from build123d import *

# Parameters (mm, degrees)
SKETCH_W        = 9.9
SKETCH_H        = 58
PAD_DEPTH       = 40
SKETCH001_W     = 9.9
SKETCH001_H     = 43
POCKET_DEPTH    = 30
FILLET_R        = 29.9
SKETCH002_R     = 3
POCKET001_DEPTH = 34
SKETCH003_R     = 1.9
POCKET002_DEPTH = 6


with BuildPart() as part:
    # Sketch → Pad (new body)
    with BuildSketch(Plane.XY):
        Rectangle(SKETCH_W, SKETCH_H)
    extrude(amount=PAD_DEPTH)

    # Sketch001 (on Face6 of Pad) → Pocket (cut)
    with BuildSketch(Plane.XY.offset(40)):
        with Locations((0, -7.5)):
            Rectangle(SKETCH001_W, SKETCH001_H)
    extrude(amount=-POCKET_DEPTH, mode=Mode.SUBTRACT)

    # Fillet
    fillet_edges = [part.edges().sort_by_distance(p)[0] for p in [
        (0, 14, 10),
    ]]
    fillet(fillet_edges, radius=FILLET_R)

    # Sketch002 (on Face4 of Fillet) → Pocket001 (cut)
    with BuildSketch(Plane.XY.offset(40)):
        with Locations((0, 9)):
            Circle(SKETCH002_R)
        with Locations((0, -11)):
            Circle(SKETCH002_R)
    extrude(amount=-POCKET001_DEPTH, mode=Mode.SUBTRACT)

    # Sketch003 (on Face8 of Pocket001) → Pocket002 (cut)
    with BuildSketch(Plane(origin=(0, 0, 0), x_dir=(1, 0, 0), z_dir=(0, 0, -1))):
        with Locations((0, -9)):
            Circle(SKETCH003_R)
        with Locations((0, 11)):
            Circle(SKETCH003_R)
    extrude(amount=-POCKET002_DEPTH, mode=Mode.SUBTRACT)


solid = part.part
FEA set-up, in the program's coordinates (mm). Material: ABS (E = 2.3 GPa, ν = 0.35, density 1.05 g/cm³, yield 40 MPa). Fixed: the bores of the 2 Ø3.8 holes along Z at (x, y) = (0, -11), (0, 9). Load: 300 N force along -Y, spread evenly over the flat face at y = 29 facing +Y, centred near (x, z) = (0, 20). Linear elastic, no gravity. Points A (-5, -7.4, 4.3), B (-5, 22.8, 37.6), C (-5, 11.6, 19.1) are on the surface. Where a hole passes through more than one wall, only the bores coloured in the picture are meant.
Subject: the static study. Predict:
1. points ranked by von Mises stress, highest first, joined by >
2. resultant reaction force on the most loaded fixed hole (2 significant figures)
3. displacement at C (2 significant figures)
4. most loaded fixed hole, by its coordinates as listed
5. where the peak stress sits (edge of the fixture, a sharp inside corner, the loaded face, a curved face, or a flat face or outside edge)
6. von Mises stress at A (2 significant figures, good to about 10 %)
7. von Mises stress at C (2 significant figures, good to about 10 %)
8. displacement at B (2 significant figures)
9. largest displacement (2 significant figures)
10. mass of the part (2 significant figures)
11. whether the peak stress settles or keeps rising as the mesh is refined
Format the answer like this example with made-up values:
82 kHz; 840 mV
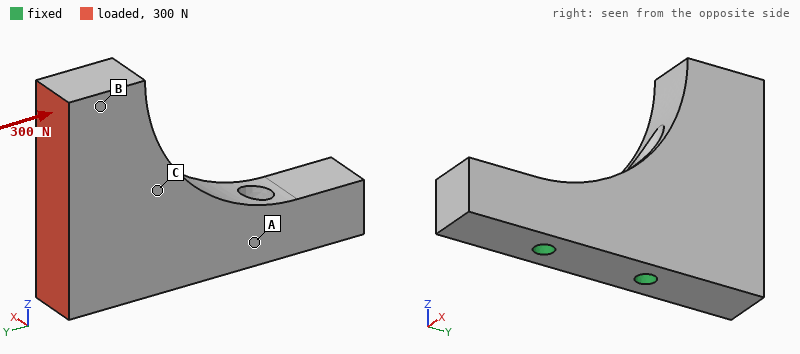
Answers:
C > A > B; 290 N; 0.097 mm; (0, -11); edge of the fixture; 3.0 MPa; 6.0 MPa; 0.28 mm; 0.32 mm; 12 g; keeps rising
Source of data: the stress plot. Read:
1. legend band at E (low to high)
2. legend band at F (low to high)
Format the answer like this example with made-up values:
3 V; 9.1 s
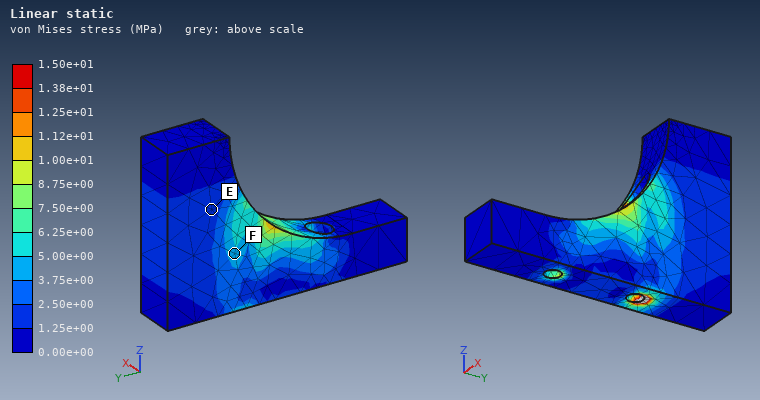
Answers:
1.25e+00 to 2.50e+00 MPa; 3.75e+00 to 5.00e+00 MPa
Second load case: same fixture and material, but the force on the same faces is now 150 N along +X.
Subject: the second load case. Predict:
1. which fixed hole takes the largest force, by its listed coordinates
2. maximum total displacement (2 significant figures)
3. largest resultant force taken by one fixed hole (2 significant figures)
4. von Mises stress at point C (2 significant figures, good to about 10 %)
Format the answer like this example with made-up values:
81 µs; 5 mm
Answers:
(0, 9); 0.77 mm; 240 N; 6.0 MPa
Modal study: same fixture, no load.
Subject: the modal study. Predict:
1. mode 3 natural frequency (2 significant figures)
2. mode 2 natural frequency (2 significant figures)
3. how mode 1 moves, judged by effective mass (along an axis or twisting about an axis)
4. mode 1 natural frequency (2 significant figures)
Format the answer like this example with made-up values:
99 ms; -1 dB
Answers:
3400 Hz; 2000 Hz; along X; 1200 Hz
